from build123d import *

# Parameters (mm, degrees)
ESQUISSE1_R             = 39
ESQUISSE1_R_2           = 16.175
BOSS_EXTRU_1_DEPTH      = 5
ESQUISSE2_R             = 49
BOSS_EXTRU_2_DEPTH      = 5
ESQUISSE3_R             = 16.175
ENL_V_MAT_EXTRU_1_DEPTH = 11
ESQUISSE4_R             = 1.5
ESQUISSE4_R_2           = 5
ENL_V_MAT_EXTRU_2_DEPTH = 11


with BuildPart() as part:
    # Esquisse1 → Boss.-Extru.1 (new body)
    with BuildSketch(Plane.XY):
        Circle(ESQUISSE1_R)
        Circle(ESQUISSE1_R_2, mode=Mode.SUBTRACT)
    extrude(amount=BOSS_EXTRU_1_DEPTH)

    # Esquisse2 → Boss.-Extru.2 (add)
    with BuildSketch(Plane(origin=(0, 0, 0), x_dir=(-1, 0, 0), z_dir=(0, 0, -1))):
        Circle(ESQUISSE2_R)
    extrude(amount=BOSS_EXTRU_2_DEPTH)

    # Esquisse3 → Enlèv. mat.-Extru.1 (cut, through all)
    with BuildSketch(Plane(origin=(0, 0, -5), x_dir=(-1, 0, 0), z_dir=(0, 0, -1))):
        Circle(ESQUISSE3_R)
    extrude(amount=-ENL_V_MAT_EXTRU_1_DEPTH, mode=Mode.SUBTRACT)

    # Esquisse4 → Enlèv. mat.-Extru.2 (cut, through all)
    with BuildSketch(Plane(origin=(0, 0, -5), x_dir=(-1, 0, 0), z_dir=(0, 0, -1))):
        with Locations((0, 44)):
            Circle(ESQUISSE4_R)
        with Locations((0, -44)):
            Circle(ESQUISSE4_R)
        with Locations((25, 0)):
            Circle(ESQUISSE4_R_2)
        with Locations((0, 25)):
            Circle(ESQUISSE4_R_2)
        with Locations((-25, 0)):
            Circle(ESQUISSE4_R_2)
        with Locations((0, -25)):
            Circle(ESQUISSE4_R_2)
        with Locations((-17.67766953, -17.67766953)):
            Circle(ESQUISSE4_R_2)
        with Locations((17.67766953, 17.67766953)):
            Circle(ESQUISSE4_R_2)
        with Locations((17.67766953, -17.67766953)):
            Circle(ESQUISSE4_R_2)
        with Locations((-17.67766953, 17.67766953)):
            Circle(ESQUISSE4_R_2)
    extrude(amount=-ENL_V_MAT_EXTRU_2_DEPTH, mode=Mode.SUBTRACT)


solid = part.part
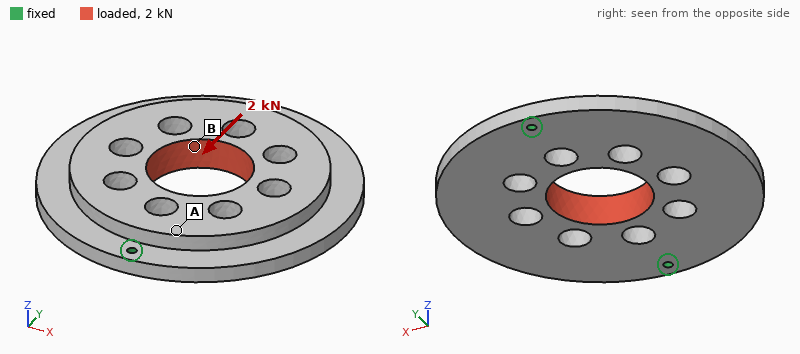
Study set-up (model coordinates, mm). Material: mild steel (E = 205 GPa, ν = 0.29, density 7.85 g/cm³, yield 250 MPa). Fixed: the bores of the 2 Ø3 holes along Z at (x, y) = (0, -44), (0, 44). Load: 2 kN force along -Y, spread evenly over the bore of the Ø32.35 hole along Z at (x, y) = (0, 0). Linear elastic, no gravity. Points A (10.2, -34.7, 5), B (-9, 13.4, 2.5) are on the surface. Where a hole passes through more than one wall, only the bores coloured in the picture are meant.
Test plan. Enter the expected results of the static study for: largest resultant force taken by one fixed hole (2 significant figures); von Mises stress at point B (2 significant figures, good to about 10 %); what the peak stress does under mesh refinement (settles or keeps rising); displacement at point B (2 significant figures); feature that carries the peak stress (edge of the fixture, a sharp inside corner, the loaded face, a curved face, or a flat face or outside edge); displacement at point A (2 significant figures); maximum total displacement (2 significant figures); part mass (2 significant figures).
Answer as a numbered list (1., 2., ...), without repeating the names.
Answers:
1. 1.0 kN
2. 4.4 MPa
3. keeps rising
4. 1.5 µm
5. edge of the fixture
6. 1.3 µm
7. 1.9 µm
8. 370 g
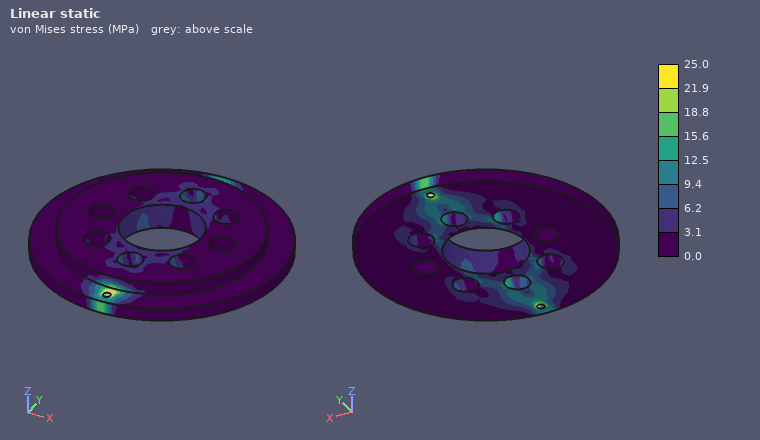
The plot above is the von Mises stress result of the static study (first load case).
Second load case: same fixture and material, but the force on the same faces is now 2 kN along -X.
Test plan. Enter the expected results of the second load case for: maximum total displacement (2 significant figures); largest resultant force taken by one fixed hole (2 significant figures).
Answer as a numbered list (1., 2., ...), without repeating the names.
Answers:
1. 17 µm
2. 1.0 kN
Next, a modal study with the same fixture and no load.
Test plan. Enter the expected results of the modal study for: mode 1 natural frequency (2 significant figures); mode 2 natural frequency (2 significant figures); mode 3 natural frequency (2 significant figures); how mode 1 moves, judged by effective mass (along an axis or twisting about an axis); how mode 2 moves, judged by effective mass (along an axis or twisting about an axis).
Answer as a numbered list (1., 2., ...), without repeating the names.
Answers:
1. 1200 Hz
2. 2300 Hz
3. 5000 Hz
4. twisting about Y
5. along Z
